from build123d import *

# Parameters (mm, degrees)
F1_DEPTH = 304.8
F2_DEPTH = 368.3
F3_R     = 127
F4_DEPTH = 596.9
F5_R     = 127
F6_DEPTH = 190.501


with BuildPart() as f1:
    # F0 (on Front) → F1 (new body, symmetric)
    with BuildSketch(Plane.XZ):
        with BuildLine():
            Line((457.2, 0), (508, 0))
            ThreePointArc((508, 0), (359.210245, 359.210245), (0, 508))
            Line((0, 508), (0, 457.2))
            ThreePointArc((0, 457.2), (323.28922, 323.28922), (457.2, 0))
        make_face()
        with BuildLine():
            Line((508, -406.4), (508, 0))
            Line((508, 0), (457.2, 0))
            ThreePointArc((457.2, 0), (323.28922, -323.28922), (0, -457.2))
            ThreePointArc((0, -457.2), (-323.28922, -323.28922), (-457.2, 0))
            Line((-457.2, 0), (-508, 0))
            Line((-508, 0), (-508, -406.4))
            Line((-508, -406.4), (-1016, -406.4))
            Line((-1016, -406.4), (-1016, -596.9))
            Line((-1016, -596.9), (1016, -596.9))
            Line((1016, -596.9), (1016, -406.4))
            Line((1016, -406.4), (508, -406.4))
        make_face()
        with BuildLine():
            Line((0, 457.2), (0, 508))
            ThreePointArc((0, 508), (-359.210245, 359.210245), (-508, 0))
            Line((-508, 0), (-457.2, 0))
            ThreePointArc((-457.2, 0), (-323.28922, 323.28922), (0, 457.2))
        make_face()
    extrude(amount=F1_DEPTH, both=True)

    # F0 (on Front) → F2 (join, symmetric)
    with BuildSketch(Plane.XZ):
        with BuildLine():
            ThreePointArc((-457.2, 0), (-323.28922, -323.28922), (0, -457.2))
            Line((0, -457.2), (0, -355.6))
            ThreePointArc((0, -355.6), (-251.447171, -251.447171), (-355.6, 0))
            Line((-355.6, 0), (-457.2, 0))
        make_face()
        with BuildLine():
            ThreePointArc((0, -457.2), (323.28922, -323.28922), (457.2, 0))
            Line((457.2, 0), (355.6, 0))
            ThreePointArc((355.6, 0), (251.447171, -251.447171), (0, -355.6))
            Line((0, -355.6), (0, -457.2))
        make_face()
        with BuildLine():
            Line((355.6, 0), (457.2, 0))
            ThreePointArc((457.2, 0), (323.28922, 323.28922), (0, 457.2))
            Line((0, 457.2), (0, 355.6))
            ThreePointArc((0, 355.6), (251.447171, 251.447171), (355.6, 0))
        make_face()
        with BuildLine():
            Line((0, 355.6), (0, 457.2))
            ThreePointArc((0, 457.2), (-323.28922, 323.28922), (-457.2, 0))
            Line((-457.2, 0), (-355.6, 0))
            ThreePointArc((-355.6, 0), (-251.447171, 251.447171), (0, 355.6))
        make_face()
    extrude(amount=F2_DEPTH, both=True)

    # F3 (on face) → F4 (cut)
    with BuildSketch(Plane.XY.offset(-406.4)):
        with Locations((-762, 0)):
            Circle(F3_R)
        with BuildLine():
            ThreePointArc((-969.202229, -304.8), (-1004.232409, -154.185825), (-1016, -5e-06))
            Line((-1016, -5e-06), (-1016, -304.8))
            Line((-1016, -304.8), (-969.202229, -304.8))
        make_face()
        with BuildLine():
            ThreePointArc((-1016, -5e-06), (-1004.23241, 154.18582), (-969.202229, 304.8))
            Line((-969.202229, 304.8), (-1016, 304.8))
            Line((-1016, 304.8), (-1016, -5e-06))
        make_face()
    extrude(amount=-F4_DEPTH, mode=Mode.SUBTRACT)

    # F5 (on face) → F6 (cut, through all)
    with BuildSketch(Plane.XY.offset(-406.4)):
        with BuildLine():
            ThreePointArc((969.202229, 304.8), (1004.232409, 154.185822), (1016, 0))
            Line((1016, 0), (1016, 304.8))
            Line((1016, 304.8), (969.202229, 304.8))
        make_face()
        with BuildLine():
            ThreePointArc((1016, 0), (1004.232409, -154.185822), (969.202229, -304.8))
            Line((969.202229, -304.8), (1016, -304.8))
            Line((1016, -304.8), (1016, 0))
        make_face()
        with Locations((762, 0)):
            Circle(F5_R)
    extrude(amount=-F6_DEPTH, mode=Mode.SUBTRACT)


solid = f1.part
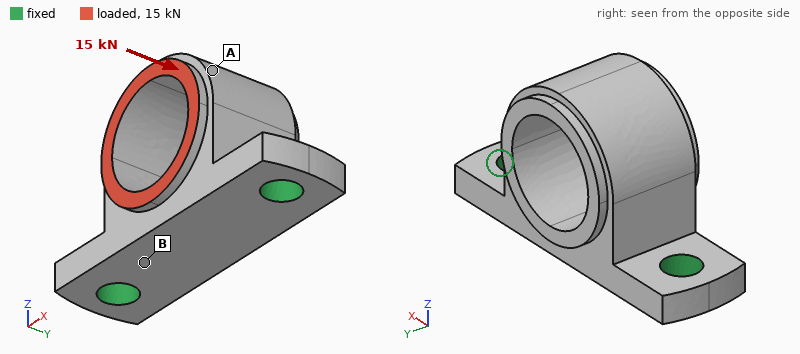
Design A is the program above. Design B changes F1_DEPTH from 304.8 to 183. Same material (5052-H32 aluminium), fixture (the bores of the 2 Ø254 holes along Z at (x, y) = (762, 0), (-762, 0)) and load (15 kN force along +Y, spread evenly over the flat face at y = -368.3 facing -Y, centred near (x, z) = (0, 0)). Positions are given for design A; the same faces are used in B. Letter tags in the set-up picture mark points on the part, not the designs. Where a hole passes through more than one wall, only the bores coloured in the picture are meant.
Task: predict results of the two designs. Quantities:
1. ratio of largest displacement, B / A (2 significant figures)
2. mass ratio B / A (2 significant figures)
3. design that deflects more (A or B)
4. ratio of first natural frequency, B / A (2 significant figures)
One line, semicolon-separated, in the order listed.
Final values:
2.2; 0.74; B; 0.73
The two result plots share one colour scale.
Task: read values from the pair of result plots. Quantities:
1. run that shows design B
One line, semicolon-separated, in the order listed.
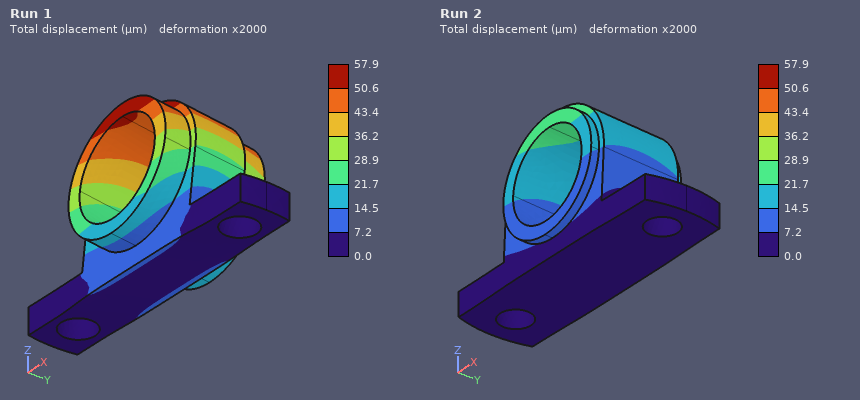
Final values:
Run 1
